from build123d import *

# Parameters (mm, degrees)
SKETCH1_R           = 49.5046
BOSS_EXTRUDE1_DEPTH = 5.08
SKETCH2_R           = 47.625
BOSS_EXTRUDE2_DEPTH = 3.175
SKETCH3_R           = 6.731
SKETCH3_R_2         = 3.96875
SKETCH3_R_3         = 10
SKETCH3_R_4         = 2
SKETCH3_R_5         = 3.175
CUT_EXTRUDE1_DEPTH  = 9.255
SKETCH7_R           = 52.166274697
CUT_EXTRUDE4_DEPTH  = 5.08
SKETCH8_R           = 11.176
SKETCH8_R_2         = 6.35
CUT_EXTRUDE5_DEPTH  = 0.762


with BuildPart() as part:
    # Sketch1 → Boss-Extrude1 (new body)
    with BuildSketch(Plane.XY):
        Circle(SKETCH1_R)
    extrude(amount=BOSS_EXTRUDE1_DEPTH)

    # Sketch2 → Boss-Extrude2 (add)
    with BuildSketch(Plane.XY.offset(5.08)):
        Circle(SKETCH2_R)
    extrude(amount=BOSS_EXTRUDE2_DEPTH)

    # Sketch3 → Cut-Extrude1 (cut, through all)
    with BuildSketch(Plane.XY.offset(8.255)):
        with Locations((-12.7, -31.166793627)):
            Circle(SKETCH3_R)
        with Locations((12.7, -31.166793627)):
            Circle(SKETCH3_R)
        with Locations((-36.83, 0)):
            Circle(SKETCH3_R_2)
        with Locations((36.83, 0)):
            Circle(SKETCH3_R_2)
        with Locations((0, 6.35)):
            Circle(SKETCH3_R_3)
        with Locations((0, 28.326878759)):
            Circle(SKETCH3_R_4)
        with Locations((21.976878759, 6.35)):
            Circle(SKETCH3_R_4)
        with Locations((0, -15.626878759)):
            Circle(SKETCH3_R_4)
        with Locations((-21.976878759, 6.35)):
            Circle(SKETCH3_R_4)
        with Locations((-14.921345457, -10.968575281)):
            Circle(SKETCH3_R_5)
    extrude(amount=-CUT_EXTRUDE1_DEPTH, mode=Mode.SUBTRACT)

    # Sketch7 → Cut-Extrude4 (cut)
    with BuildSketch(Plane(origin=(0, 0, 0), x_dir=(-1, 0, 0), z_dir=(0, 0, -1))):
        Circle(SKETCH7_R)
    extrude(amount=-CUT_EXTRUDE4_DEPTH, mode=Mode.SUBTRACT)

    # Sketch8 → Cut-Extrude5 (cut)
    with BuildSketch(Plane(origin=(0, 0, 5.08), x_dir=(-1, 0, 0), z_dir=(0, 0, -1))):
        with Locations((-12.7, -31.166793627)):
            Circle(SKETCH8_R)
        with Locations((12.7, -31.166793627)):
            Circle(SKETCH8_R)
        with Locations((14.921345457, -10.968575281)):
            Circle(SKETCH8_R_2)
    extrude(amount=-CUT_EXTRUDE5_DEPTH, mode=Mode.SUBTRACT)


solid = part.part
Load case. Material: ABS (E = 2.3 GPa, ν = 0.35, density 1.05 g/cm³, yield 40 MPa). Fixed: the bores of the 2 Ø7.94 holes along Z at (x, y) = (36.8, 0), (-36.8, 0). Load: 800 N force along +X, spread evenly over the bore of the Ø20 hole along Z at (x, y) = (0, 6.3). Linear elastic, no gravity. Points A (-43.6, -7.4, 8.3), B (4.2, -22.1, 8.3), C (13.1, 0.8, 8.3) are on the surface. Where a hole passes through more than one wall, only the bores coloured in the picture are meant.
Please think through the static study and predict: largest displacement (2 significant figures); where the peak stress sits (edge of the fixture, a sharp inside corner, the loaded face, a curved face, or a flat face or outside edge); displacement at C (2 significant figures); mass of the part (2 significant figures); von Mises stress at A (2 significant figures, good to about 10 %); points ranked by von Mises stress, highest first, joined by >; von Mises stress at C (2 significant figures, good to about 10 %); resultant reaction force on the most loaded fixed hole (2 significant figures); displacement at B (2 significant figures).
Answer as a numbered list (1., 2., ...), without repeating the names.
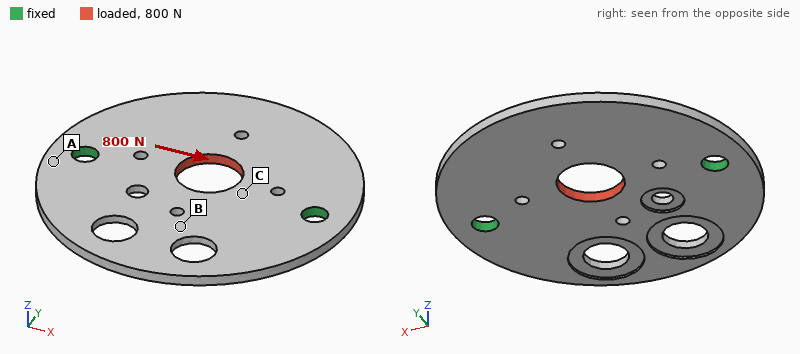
1. 93 µm
2. a curved face
3. 52 µm
4. 21 g
5. 1.9 MPa
6. C > A > B
7. 5.0 MPa
8. 410 N
9. 30 µm
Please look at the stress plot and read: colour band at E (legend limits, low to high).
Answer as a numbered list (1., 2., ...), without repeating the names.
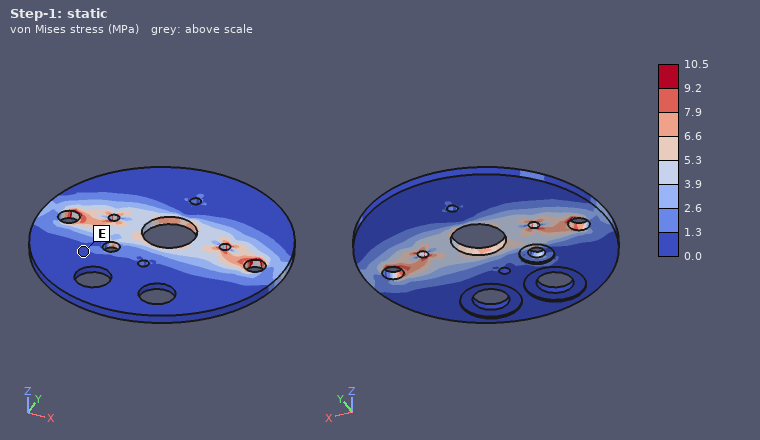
1. 0.0 to 1.3 MPa
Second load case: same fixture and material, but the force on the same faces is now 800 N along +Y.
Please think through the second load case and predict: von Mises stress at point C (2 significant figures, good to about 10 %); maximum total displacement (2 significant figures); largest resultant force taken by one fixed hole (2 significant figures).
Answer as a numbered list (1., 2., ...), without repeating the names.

1. 3.8 MPa
2. 0.12 mm
3. 400 N
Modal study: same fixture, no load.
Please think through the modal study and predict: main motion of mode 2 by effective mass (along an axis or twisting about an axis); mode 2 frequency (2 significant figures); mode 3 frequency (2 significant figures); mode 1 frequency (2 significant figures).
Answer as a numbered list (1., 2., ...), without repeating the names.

1. along Z
2. 420 Hz
3. 900 Hz
4. 340 Hz
